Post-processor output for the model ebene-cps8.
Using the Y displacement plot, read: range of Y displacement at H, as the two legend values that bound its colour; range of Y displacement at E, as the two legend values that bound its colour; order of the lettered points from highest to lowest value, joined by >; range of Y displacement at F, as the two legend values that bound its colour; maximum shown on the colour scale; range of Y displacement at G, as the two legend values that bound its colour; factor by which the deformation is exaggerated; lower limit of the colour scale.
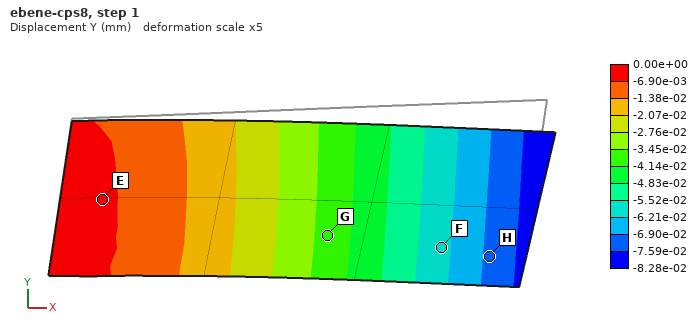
-7.59e-02 to -6.90e-02 mm
-6.90e-03 to 0.00e+00 mm
E > G > F > H
-6.21e-02 to -5.52e-02 mm
0.00e+00 mm
-4.14e-02 to -3.45e-02 mm
5
-8.28e-02 mm
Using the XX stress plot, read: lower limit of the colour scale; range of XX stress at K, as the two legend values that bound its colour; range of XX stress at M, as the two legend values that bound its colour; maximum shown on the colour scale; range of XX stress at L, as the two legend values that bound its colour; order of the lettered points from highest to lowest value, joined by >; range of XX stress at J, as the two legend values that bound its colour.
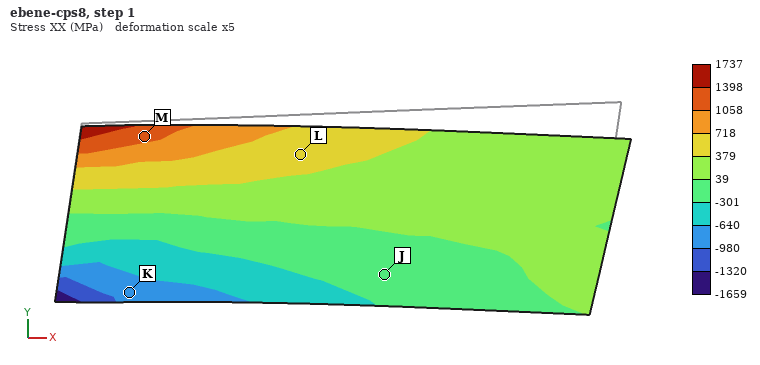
-1659 MPa
-980 to -640 MPa
1058 to 1398 MPa
1737 MPa
379 to 718 MPa
M > L > J > K
-301 to 39 MPa
